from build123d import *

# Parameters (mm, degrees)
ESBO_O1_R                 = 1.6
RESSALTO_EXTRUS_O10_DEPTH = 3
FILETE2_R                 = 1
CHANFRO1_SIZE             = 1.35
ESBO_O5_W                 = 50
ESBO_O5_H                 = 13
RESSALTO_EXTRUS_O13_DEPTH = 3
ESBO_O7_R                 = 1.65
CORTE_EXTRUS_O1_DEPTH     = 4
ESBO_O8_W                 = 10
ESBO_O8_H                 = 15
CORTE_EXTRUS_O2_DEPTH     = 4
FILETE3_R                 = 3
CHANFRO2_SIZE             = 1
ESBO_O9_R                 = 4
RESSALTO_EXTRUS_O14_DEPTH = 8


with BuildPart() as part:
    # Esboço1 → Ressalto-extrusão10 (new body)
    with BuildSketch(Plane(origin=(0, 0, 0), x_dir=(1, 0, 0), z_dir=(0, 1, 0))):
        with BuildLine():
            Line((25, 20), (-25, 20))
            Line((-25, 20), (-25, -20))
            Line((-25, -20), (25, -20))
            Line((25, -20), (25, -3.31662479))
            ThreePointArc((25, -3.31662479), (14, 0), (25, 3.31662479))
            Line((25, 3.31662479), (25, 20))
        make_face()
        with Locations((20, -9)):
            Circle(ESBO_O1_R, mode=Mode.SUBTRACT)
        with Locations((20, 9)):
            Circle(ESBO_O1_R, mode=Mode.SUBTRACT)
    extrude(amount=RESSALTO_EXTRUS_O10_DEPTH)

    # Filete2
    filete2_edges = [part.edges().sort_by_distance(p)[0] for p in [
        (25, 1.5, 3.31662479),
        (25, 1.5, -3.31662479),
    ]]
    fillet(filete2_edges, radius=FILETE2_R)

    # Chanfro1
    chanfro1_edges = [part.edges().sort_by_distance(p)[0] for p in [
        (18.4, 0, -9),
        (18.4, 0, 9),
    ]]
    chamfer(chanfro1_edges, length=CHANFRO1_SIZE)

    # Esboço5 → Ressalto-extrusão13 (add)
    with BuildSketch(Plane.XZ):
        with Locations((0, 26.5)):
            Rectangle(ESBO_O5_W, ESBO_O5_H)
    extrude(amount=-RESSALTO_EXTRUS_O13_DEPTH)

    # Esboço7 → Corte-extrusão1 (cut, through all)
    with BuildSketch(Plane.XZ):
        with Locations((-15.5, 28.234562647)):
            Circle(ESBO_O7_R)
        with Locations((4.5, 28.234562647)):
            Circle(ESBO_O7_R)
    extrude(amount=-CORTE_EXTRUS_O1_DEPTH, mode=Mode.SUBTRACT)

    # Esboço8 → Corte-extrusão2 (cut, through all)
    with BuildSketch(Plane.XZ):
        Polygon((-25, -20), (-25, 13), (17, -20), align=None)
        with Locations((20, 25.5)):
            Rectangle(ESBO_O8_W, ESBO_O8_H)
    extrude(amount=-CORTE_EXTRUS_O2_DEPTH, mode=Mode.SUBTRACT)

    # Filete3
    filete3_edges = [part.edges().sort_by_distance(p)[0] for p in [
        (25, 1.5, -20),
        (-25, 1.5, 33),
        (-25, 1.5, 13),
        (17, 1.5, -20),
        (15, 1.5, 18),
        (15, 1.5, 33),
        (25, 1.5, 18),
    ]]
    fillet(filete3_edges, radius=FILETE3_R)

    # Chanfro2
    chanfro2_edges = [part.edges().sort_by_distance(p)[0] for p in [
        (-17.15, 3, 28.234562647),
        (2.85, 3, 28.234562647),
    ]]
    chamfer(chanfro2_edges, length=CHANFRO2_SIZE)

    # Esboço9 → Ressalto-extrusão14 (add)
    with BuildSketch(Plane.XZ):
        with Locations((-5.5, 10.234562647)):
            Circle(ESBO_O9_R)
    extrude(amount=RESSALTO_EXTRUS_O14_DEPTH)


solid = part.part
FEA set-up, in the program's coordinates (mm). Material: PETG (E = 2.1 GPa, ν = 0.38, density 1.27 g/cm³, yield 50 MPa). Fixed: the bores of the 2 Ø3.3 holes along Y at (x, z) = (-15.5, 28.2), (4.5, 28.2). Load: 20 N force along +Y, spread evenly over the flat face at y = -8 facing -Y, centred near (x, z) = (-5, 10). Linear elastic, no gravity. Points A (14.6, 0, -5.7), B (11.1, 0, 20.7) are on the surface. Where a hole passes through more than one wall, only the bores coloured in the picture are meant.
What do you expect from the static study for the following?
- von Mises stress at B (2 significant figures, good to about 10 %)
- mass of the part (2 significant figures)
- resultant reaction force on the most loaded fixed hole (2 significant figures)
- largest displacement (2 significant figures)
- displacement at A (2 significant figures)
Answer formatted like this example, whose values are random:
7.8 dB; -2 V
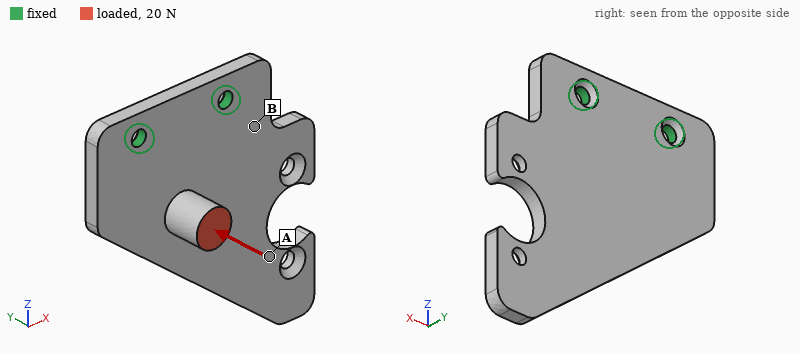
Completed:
3.2 MPa; 6.8 g; 10 N; 0.88 mm; 0.58 mm
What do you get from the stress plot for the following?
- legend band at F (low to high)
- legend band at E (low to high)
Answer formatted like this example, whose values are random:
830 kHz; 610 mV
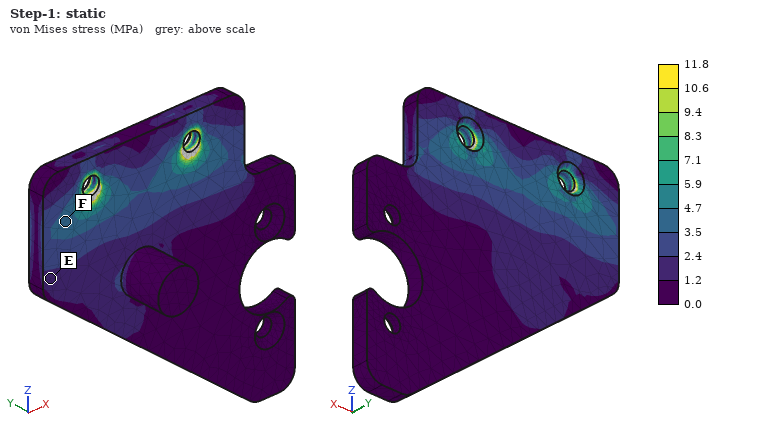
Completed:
3.5 to 4.7 MPa; 1.2 to 2.4 MPa
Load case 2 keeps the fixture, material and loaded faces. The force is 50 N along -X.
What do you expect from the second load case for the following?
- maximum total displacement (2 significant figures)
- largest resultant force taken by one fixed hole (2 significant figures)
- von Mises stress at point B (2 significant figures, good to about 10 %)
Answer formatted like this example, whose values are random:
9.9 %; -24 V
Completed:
0.75 mm; 51 N; 2.1 MPa
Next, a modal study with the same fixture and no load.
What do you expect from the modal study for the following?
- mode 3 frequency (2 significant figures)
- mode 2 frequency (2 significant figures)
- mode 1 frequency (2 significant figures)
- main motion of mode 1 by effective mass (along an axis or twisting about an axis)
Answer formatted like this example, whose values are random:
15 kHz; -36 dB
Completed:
1300 Hz; 970 Hz; 320 Hz; along Y
